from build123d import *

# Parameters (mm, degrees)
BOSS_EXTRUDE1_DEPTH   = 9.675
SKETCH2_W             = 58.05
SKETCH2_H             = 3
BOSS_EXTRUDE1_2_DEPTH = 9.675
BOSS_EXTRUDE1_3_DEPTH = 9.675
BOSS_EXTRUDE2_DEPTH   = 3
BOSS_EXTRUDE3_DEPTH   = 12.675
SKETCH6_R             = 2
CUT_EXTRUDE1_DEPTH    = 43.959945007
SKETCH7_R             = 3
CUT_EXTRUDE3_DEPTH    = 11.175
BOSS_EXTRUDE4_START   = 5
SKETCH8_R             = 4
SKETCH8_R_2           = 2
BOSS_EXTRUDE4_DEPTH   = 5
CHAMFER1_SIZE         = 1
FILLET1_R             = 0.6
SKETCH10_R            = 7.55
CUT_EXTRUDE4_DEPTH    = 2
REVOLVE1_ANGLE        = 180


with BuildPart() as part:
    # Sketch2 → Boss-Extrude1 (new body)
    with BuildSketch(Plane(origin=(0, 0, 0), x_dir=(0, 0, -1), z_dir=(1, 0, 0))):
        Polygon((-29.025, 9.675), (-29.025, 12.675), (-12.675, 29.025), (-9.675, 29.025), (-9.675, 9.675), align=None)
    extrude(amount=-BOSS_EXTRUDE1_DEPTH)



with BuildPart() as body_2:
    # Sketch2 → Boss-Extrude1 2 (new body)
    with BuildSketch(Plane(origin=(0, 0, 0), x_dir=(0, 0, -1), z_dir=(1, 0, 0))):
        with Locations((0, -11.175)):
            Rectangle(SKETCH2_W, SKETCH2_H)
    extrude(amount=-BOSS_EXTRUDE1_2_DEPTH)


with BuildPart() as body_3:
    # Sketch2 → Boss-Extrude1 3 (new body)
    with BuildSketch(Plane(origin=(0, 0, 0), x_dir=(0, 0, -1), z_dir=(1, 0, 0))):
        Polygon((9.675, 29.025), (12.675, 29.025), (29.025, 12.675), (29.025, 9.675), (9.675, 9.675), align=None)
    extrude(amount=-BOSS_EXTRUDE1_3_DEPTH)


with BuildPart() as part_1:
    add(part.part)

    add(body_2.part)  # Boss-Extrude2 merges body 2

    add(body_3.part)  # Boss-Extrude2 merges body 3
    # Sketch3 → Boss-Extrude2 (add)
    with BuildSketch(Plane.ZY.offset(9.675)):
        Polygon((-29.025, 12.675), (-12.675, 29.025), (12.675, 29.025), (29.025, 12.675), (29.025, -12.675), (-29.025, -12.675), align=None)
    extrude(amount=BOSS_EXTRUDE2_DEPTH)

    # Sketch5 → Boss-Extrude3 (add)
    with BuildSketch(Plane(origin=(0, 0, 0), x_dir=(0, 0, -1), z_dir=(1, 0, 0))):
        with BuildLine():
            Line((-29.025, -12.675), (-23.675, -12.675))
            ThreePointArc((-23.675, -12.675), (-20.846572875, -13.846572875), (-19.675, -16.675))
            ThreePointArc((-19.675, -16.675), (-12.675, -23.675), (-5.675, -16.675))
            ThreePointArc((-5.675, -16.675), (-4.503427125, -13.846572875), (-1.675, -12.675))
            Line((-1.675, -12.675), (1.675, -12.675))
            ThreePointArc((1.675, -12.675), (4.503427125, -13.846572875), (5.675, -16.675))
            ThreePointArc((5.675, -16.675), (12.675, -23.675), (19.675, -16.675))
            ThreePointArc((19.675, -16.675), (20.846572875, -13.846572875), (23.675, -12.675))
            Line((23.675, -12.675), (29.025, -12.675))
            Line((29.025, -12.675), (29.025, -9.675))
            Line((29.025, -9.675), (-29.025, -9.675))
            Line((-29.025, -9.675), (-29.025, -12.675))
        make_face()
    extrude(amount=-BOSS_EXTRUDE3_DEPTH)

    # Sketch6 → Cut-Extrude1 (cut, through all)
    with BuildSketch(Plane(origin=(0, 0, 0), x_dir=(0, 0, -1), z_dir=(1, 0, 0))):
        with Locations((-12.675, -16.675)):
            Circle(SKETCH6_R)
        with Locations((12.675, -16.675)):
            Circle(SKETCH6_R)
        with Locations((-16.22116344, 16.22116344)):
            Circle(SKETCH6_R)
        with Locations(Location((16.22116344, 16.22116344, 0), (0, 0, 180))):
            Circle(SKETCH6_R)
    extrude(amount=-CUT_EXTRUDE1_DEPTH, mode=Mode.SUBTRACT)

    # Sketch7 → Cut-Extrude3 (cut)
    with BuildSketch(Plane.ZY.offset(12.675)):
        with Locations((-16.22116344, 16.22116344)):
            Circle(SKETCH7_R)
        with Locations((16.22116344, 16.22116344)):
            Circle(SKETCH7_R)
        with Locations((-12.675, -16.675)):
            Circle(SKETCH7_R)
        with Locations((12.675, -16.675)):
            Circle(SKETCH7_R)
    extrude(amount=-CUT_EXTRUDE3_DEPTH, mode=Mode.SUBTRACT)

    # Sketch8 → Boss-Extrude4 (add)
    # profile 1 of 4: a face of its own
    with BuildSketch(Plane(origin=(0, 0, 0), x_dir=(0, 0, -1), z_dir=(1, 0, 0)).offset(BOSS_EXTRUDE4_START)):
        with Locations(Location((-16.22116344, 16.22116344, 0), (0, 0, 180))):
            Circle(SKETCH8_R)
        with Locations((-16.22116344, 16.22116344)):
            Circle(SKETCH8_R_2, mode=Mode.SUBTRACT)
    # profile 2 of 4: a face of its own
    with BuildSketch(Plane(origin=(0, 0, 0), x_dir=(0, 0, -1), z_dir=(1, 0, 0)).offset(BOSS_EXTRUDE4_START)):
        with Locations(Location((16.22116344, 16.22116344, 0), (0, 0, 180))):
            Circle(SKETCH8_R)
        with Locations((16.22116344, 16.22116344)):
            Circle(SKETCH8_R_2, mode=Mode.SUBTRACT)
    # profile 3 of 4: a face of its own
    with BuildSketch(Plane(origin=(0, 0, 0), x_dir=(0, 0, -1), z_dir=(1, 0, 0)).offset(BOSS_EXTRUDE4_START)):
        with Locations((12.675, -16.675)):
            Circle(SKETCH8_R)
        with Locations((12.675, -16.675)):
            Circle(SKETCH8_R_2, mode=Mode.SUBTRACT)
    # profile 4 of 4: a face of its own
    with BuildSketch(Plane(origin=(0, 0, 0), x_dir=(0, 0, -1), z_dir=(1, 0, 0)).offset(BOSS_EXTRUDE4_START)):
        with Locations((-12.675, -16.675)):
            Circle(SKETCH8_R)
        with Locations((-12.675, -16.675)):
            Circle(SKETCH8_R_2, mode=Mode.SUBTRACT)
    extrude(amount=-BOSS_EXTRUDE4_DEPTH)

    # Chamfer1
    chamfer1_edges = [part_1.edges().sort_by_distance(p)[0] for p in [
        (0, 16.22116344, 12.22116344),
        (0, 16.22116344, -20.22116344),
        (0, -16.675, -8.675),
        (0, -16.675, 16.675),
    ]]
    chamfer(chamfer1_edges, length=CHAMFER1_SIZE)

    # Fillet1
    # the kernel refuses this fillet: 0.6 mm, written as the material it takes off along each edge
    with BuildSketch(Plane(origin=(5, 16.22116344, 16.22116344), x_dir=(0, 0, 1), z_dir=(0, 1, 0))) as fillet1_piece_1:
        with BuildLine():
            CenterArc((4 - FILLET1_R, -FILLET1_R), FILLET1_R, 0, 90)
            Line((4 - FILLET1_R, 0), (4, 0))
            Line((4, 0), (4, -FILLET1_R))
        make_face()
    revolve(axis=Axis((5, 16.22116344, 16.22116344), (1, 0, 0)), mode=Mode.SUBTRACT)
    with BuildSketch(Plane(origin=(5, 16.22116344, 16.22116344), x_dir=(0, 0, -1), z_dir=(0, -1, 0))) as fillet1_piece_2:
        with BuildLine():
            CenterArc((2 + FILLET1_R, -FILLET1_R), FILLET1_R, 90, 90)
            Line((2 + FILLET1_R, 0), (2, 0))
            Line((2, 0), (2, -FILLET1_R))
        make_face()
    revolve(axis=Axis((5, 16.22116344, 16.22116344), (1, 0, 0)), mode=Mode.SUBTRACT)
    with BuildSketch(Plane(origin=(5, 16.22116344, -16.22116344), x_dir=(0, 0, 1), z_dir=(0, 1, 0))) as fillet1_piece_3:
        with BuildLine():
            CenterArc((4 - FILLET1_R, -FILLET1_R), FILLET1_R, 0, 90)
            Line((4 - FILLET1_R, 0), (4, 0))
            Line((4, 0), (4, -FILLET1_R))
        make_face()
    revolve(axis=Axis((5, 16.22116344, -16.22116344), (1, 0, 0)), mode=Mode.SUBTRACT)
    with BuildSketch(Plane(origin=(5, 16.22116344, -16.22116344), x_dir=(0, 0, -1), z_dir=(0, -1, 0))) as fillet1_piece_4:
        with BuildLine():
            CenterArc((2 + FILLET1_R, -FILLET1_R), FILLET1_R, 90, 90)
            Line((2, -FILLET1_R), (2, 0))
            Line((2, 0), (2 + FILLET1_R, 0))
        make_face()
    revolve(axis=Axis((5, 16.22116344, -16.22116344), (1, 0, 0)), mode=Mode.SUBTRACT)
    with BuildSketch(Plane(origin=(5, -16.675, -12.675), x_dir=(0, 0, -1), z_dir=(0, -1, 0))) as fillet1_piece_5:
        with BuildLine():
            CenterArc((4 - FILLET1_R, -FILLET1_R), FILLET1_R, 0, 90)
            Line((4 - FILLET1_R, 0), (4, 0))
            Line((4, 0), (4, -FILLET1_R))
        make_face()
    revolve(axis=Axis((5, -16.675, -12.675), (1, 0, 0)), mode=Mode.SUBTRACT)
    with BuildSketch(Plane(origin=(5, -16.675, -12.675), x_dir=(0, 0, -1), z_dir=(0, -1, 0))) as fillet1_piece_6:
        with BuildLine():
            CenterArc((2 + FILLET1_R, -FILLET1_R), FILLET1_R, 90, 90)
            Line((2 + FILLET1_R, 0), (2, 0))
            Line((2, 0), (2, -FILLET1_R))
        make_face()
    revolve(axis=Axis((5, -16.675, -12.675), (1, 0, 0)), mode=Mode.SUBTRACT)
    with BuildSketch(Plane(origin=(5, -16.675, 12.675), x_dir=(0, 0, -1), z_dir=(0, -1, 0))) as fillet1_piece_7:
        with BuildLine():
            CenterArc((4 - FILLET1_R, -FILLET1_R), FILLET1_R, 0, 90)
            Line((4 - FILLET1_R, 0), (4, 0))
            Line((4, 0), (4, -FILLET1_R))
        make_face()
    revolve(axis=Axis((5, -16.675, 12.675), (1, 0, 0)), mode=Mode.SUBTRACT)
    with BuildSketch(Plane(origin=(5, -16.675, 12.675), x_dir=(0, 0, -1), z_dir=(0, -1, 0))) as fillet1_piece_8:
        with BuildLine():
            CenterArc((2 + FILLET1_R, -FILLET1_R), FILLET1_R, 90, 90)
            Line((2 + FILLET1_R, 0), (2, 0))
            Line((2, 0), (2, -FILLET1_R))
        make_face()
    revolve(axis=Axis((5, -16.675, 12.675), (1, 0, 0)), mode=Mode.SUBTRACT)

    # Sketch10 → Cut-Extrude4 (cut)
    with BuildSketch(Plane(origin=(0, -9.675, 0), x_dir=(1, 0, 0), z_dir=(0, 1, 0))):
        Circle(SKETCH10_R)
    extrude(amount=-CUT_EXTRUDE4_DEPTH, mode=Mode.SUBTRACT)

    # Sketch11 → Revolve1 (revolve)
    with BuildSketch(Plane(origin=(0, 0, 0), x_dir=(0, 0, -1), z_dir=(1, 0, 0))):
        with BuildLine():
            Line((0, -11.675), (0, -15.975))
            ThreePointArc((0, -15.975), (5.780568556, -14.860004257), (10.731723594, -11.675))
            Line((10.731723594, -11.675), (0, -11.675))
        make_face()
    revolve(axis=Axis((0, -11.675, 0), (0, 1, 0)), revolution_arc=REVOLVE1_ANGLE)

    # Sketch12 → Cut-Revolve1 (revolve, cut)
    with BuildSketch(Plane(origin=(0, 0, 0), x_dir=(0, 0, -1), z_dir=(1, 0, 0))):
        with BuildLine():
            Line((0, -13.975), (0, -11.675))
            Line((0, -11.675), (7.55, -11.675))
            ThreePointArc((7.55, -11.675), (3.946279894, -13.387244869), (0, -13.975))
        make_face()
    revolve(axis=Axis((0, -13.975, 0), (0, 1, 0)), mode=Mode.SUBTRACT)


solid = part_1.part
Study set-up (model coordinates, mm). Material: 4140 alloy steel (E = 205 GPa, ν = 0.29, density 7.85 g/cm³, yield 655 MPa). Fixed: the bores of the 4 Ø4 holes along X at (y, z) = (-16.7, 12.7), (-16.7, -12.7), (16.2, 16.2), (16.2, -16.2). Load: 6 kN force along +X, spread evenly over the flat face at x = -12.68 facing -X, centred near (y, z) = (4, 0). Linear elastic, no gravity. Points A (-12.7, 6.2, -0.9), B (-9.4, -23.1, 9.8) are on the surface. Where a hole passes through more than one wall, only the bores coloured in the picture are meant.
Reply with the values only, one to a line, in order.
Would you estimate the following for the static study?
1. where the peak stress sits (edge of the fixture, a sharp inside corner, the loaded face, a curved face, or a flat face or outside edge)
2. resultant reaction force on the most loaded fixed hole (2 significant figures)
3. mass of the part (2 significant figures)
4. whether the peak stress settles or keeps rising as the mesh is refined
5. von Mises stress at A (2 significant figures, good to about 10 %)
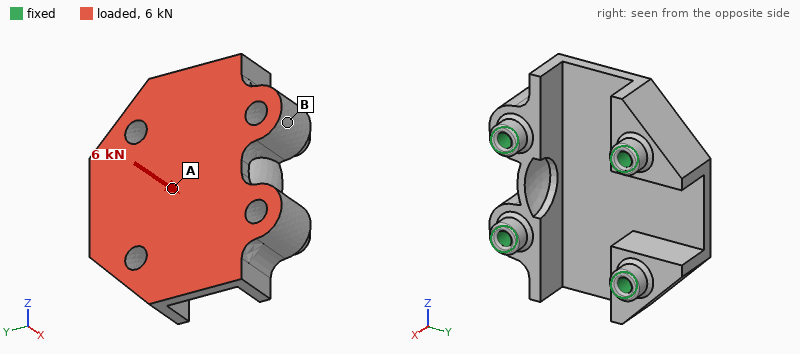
edge of the fixture
1.9 kN
120 g
keeps rising
34 MPa
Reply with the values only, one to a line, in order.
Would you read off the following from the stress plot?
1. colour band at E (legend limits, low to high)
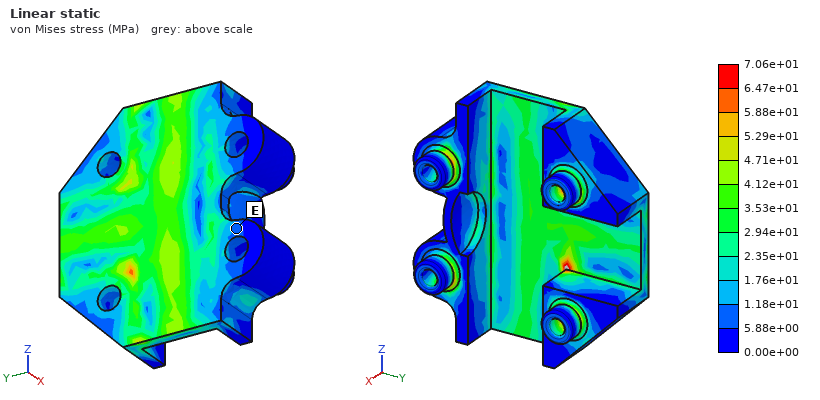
5.88e+00 to 1.18e+01 MPa
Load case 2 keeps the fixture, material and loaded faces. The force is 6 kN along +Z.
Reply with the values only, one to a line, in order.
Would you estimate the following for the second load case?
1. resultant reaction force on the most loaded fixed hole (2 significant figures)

2.2 kN
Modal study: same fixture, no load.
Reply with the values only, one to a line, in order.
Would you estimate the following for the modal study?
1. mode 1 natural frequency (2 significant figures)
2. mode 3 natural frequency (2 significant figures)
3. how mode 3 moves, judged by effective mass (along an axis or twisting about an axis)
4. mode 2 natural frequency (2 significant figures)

12 kHz
15 kHz
along Z
12 kHz
